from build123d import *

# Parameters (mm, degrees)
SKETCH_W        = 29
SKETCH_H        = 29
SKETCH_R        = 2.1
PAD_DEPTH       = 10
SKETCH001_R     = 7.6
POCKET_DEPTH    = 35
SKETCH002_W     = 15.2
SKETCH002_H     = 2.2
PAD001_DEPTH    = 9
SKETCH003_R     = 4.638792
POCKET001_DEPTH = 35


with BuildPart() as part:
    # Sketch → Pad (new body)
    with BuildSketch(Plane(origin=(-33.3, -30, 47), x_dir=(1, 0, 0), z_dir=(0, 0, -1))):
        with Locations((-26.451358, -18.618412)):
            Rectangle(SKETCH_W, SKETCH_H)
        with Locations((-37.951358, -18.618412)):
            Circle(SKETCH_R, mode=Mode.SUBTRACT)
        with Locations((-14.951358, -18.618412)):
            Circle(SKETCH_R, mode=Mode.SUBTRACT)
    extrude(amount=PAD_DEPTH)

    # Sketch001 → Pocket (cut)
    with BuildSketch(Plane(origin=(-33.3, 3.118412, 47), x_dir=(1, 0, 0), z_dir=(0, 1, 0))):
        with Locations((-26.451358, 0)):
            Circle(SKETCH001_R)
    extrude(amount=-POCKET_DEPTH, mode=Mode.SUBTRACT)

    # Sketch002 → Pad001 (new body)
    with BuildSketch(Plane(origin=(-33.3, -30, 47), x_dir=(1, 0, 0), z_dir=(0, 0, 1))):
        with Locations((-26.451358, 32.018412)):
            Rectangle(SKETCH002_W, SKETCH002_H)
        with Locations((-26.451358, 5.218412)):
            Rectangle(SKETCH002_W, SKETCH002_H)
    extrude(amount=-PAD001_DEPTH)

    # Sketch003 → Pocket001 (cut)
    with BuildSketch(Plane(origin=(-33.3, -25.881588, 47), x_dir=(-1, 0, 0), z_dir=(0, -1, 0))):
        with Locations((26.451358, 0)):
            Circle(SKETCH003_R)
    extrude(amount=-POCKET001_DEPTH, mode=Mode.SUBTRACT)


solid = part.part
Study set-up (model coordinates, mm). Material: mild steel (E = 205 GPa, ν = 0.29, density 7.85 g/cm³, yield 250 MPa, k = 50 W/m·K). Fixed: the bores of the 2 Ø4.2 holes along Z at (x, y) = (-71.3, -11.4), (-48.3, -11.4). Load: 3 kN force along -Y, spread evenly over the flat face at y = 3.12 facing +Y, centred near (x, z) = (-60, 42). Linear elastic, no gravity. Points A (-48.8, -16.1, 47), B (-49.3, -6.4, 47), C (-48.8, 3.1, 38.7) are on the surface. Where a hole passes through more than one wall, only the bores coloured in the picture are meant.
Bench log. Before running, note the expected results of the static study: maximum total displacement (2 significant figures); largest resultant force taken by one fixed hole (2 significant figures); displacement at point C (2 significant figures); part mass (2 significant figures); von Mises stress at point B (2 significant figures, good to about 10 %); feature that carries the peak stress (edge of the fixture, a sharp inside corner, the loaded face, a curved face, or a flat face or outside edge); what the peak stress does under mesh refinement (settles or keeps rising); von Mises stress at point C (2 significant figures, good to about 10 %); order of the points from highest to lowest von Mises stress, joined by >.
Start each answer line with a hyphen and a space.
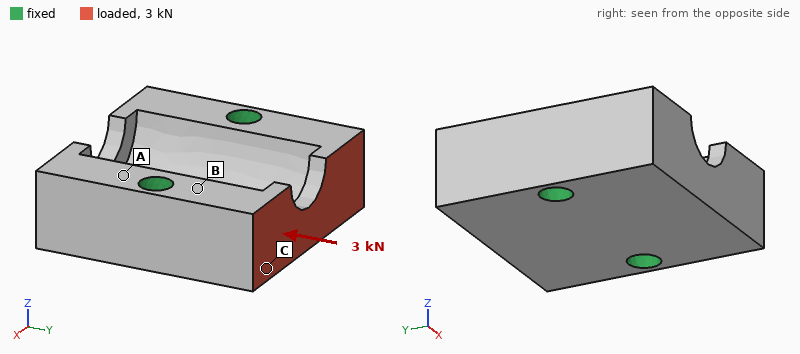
- 3.8 µm
- 1.5 kN
- 0.88 µm
- 45 g
- 22 MPa
- a sharp inside corner
- keeps rising
- 12 MPa
- B > C > A
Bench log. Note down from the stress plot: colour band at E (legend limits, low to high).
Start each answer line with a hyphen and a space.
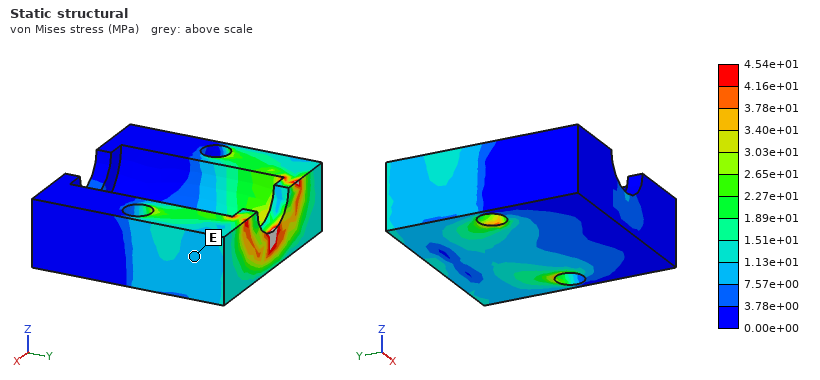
- 7.57e+00 to 1.13e+01 MPa
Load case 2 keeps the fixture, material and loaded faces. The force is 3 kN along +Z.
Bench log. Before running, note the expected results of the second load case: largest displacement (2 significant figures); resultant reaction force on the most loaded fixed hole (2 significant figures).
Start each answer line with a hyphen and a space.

- 16 µm
- 1.5 kN
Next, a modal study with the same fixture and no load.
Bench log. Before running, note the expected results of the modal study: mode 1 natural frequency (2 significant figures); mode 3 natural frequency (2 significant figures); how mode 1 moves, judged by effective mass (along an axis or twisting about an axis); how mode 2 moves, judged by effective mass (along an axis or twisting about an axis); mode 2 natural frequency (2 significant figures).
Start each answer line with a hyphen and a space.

- 27 kHz
- 32 kHz
- twisting about X
- along Z
- 30 kHz
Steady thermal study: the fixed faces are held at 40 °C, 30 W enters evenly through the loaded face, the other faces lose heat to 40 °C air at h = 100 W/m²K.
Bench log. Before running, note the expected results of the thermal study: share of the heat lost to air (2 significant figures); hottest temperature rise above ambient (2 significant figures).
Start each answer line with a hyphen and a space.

- 9.5 %
- 46 K
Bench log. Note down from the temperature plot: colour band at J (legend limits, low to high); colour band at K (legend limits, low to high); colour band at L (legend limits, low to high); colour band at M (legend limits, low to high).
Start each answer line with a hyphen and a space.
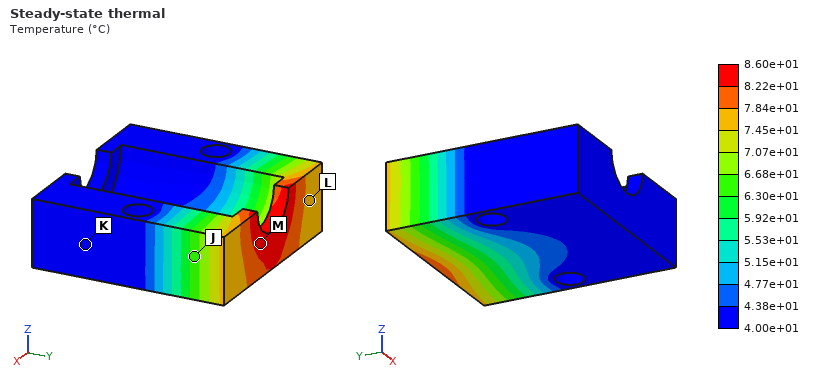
- 6.30e+01 to 6.68e+01 °C
- 4.00e+01 to 4.38e+01 °C
- 7.45e+01 to 7.84e+01 °C
- 8.22e+01 to 8.60e+01 °C
